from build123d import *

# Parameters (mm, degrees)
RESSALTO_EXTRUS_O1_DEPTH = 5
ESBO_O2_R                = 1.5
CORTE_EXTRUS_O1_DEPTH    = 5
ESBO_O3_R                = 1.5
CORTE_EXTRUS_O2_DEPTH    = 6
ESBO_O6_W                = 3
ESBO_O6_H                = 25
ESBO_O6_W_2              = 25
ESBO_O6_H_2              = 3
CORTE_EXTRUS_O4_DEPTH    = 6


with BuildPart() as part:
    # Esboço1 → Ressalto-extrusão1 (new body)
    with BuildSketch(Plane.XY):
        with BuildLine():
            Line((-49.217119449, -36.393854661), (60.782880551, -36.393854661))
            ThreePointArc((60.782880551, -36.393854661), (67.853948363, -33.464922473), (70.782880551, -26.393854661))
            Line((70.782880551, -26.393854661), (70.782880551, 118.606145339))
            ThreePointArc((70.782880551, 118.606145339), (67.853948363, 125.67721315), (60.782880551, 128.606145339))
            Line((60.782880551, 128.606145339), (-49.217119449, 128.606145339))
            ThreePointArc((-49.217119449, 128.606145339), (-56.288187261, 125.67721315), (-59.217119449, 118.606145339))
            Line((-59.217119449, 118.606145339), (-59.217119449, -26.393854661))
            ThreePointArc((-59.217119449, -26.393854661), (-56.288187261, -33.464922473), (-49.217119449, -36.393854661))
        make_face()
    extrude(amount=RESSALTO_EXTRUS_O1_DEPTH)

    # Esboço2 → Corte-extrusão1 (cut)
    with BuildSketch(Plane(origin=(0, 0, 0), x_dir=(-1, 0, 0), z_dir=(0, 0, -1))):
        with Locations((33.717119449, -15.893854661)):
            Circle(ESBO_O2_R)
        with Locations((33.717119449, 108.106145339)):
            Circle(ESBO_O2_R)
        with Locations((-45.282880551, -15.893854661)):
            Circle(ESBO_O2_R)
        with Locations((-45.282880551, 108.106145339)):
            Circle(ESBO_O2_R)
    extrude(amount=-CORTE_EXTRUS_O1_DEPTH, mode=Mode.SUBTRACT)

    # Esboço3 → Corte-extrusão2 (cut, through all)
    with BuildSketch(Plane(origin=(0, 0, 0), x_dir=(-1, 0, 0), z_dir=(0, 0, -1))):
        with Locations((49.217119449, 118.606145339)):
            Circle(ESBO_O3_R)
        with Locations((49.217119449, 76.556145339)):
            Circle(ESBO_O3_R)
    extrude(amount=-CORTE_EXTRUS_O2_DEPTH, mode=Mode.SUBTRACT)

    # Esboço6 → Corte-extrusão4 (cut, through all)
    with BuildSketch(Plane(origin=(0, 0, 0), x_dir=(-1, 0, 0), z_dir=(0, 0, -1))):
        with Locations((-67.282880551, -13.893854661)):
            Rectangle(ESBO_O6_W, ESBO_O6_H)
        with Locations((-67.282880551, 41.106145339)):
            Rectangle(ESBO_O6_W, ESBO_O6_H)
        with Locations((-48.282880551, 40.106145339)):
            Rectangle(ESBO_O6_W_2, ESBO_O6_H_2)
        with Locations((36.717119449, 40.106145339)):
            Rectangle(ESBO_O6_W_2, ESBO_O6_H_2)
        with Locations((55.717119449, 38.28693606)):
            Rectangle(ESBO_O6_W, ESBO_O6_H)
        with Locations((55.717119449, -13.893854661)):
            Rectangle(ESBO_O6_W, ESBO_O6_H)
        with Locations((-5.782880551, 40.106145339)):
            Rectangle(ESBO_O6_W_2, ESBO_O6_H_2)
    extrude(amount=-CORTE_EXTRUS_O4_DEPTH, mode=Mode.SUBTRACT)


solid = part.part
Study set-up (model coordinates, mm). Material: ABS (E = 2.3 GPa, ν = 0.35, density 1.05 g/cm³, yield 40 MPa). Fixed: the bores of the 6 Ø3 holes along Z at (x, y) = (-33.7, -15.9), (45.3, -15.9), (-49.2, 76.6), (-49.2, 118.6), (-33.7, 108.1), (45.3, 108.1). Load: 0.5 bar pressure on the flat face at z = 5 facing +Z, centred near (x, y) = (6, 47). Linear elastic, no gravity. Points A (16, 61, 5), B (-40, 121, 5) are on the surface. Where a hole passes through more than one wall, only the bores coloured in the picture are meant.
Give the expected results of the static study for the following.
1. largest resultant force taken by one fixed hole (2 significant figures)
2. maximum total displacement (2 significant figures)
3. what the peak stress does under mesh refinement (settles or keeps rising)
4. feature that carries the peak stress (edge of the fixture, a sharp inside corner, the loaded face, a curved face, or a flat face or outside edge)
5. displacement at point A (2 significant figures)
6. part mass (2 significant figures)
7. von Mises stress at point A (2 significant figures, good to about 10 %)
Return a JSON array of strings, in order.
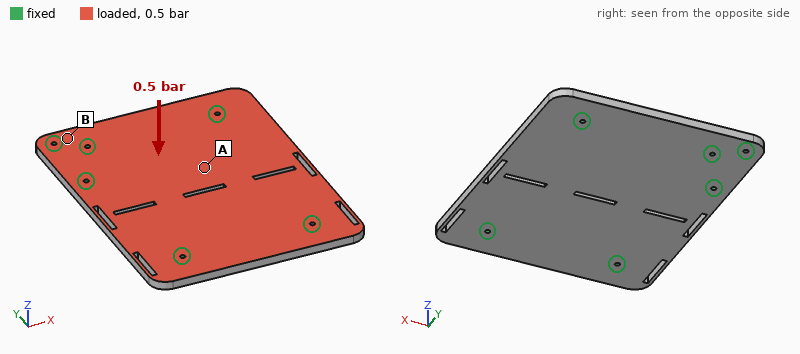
["260 N", "2.3 mm", "keeps rising", "edge of the fixture", "1.7 mm", "110 g", "5.3 MPa"]
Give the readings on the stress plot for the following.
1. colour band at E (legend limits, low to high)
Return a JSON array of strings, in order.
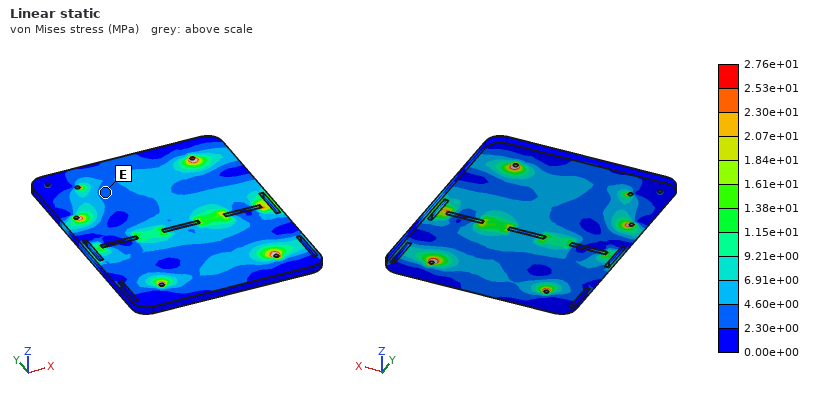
["2.30e+00 to 4.60e+00 MPa"]
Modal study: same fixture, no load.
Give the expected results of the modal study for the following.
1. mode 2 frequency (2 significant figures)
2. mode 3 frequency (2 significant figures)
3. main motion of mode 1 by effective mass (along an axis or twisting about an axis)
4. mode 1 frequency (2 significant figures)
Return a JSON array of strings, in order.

["620 Hz", "830 Hz", "along Z", "390 Hz"]
